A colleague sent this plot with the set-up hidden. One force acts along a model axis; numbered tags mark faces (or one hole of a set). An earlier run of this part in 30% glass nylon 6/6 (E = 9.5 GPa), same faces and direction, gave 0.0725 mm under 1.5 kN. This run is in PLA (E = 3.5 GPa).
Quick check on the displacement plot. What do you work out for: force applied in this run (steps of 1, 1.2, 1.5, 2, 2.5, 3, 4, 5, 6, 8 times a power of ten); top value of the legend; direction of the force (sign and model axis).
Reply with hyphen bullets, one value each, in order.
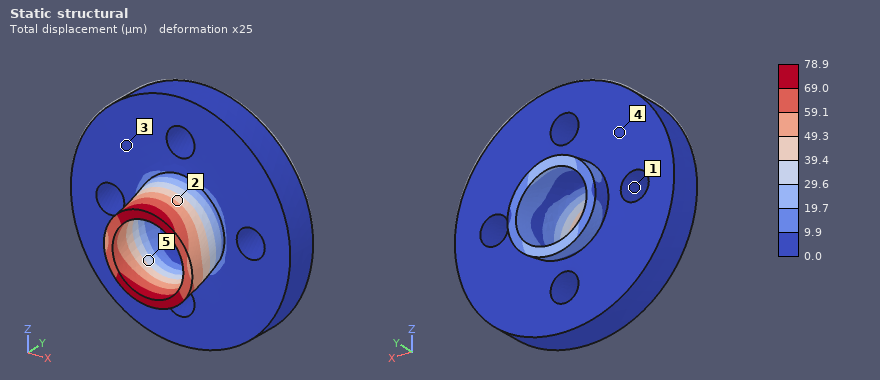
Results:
- 600 N
- 78.9 µm
- -Z
